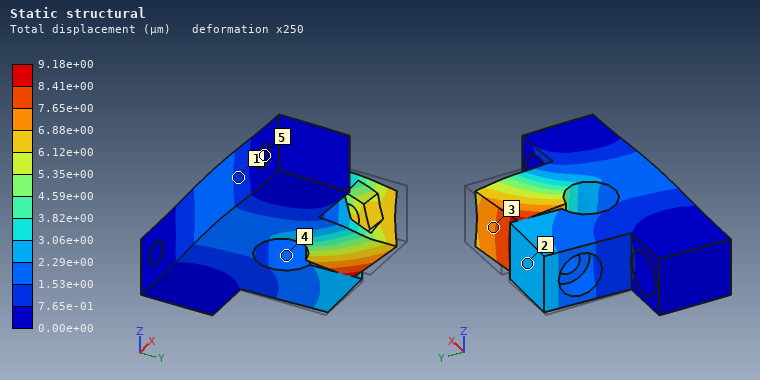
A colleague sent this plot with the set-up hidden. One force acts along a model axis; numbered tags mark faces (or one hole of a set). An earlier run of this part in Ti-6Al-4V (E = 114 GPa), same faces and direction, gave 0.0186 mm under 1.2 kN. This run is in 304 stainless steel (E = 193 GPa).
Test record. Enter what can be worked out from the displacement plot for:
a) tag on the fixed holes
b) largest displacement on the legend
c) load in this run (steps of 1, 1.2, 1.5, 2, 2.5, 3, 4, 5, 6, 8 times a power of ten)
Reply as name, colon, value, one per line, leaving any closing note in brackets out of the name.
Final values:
tag on the fixed holes: 5
largest displacement on the legend: 9.18e+00 µm
load in this run: 1 kN
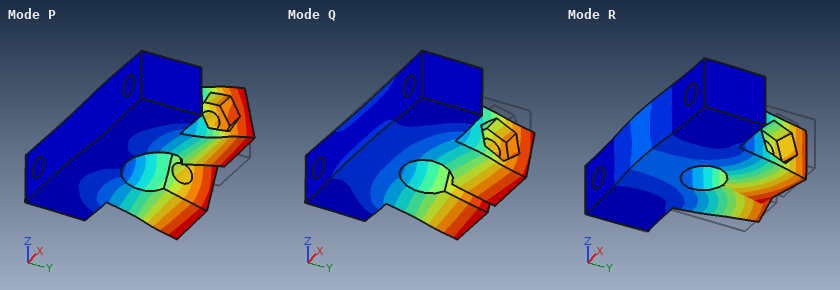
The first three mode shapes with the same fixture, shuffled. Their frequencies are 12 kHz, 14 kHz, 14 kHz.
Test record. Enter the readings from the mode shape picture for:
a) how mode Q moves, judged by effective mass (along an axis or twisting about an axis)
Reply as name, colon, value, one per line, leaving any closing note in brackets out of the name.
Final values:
how mode Q moves, judged by effective mass: along Z
